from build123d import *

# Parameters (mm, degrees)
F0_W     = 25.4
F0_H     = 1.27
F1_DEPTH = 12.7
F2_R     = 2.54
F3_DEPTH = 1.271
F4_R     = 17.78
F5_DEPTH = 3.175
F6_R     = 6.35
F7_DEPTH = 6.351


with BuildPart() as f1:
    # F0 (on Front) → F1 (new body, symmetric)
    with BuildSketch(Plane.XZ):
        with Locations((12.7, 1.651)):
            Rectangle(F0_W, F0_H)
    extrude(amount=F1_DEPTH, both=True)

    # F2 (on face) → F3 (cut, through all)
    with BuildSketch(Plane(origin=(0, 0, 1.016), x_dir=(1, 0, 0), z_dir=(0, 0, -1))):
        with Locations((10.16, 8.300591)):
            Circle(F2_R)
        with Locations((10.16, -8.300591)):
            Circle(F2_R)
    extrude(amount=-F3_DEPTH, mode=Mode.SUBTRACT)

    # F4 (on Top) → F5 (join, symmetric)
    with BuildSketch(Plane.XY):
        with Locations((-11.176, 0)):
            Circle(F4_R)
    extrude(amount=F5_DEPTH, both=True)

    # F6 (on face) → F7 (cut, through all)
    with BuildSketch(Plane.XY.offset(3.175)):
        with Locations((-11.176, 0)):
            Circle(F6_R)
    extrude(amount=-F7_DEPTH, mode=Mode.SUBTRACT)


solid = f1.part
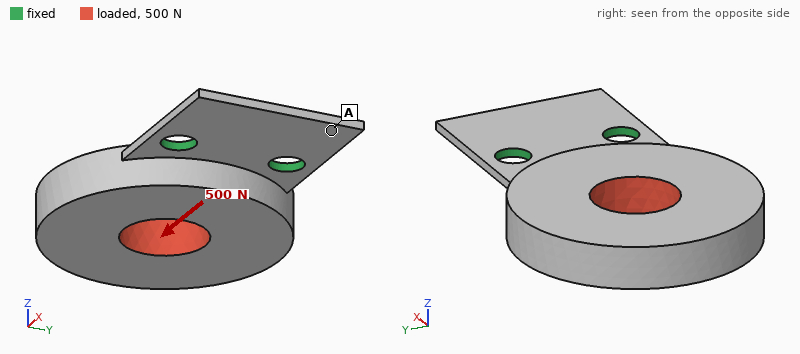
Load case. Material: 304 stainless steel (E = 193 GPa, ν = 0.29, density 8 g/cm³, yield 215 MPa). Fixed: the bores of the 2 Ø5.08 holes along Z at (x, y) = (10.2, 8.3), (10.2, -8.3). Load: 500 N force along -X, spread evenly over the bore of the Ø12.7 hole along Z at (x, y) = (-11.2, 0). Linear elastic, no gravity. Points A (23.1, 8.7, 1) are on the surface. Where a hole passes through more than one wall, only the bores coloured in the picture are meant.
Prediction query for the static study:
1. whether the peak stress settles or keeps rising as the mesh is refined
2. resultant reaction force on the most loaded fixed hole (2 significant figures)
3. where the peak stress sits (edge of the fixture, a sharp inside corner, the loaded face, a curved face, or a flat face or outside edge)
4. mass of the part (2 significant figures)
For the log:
keeps rising
250 N
edge of the fixture
49 g
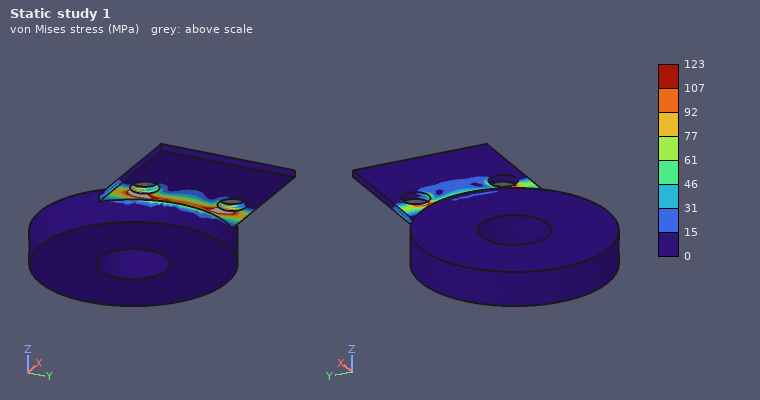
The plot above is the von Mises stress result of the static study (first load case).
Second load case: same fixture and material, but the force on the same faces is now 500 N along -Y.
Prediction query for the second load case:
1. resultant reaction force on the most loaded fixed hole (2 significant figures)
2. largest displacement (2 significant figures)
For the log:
610 N
9.5 µm
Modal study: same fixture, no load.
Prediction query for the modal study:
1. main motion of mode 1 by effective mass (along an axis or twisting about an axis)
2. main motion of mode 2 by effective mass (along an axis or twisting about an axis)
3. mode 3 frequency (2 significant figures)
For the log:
along Z
twisting about X
5500 Hz
